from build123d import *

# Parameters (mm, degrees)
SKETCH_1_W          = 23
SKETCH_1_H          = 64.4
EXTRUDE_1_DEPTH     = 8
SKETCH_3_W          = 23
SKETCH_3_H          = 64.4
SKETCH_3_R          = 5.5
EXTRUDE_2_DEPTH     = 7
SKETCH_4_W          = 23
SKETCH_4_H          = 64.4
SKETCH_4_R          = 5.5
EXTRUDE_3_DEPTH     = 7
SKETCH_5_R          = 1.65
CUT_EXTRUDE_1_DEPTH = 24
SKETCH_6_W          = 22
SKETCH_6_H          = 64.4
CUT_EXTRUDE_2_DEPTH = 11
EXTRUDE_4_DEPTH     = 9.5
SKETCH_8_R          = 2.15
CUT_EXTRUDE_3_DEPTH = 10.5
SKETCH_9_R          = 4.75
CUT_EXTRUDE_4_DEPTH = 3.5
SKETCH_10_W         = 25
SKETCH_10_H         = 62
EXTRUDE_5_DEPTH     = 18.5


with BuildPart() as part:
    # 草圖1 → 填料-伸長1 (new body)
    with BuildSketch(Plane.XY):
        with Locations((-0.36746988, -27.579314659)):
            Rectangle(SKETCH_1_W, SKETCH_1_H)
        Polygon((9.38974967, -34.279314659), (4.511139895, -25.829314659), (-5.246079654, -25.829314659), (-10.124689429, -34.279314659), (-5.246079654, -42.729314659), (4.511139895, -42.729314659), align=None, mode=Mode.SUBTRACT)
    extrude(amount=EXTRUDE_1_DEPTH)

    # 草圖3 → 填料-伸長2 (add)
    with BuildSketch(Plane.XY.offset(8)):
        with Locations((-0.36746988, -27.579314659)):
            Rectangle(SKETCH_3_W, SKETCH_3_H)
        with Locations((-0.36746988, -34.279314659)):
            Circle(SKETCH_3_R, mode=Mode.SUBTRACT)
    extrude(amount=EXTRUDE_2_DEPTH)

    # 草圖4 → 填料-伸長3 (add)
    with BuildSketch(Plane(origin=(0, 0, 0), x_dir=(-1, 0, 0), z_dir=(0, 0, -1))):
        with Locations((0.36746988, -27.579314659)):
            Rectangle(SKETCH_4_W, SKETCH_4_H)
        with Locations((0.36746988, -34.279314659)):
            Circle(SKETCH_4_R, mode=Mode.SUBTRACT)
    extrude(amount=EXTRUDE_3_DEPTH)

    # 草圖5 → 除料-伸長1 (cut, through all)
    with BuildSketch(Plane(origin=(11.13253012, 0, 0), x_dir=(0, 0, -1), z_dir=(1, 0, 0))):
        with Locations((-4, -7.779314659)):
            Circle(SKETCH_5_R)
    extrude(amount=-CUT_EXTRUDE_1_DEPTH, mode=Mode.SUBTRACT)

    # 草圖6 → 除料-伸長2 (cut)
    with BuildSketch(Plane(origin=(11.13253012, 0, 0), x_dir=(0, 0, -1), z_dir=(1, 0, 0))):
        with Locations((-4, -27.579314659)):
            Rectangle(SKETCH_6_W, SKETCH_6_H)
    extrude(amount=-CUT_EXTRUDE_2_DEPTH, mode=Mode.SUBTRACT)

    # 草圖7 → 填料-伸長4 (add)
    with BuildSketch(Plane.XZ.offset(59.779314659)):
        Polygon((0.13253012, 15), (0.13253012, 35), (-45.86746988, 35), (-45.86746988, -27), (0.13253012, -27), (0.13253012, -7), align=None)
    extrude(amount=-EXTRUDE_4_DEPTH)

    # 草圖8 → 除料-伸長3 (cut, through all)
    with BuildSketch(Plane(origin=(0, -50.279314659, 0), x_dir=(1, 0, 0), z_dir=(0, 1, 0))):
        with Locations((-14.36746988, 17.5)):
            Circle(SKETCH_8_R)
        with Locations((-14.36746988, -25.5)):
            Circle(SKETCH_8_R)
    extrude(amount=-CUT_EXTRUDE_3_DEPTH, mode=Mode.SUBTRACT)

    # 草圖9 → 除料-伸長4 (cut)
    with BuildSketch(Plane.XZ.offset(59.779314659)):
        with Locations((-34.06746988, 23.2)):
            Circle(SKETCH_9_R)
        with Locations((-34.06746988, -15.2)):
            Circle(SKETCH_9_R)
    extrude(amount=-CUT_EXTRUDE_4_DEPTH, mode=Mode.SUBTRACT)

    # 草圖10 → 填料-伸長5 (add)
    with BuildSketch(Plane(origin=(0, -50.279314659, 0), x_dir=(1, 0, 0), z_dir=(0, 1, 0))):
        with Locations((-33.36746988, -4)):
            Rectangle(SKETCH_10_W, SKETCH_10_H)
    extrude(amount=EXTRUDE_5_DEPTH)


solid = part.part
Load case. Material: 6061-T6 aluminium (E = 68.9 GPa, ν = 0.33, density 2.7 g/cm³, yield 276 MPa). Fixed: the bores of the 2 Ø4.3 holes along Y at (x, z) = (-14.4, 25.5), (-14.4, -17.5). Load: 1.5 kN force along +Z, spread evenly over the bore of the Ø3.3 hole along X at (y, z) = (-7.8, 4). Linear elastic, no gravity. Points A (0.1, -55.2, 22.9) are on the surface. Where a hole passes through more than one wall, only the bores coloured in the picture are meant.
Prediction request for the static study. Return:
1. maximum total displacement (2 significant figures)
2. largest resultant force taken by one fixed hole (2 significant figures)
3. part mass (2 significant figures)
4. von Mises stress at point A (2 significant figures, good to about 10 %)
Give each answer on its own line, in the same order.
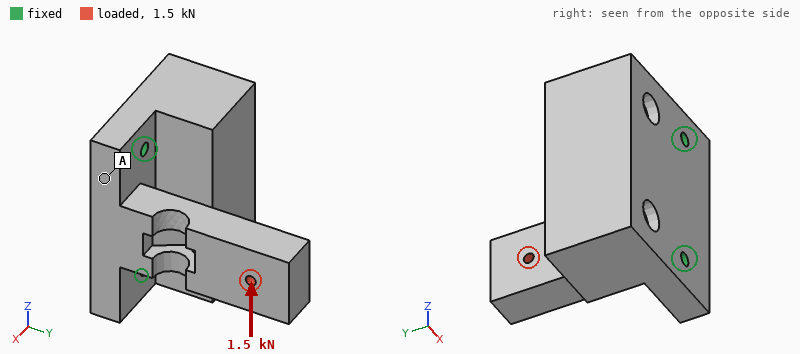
0.22 mm
2.1 kN
180 g
17 MPa
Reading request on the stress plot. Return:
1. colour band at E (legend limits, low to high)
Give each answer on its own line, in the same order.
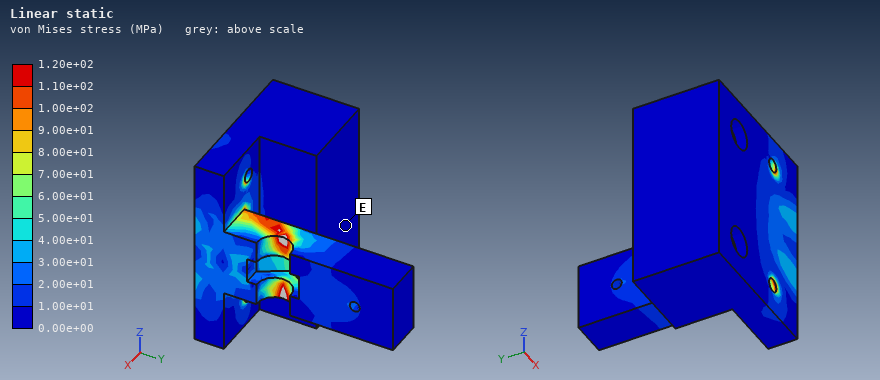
0.00e+00 to 1.00e+01 MPa
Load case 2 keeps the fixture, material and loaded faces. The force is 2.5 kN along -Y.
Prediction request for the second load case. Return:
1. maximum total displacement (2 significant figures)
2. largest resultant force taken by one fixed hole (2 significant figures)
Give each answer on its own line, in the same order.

0.21 mm
1.3 kN
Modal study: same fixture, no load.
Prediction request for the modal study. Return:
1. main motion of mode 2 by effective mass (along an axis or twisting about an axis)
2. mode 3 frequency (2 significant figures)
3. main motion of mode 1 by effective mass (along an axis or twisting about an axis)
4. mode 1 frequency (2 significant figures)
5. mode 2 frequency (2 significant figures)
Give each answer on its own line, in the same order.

along Y
3400 Hz
along X
1500 Hz
3200 Hz
